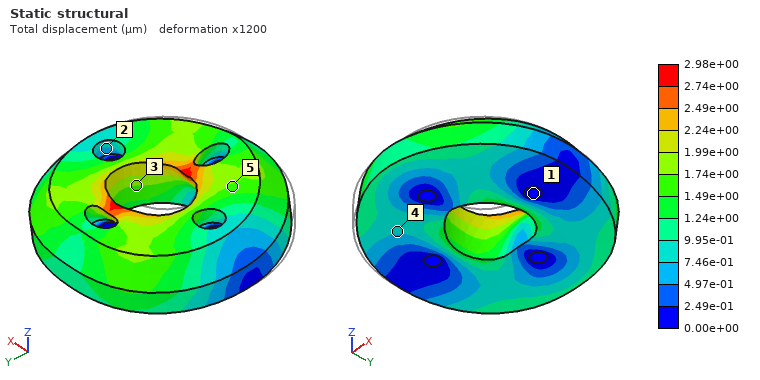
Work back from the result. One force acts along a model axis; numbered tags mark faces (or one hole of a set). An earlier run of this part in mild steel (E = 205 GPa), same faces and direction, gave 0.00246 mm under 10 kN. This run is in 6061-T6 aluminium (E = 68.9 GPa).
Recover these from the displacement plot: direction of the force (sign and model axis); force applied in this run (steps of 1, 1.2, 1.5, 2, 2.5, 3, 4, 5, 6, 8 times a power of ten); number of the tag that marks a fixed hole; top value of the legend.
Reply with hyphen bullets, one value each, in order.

- +Y
- 4 kN
- 1
- 2.98e+00 µm
